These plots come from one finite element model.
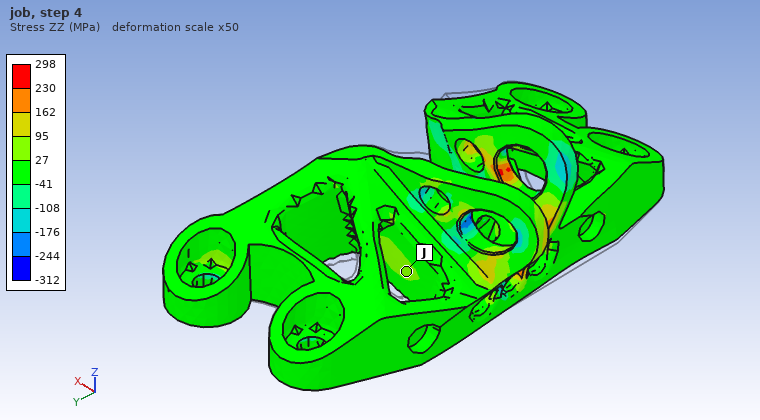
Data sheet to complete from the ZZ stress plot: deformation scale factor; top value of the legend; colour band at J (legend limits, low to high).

50
298 MPa
27 to 95 MPa
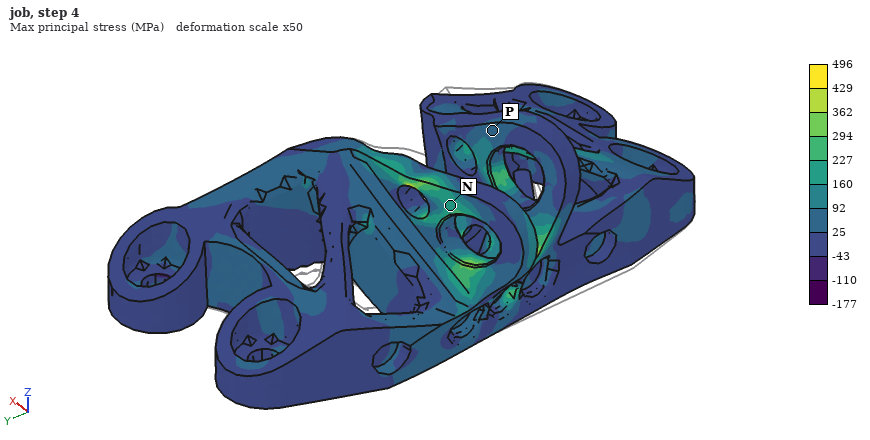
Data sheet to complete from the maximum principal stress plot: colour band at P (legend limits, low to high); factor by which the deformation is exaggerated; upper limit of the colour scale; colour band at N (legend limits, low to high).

25 to 92 MPa
50
496 MPa
160 to 227 MPa
